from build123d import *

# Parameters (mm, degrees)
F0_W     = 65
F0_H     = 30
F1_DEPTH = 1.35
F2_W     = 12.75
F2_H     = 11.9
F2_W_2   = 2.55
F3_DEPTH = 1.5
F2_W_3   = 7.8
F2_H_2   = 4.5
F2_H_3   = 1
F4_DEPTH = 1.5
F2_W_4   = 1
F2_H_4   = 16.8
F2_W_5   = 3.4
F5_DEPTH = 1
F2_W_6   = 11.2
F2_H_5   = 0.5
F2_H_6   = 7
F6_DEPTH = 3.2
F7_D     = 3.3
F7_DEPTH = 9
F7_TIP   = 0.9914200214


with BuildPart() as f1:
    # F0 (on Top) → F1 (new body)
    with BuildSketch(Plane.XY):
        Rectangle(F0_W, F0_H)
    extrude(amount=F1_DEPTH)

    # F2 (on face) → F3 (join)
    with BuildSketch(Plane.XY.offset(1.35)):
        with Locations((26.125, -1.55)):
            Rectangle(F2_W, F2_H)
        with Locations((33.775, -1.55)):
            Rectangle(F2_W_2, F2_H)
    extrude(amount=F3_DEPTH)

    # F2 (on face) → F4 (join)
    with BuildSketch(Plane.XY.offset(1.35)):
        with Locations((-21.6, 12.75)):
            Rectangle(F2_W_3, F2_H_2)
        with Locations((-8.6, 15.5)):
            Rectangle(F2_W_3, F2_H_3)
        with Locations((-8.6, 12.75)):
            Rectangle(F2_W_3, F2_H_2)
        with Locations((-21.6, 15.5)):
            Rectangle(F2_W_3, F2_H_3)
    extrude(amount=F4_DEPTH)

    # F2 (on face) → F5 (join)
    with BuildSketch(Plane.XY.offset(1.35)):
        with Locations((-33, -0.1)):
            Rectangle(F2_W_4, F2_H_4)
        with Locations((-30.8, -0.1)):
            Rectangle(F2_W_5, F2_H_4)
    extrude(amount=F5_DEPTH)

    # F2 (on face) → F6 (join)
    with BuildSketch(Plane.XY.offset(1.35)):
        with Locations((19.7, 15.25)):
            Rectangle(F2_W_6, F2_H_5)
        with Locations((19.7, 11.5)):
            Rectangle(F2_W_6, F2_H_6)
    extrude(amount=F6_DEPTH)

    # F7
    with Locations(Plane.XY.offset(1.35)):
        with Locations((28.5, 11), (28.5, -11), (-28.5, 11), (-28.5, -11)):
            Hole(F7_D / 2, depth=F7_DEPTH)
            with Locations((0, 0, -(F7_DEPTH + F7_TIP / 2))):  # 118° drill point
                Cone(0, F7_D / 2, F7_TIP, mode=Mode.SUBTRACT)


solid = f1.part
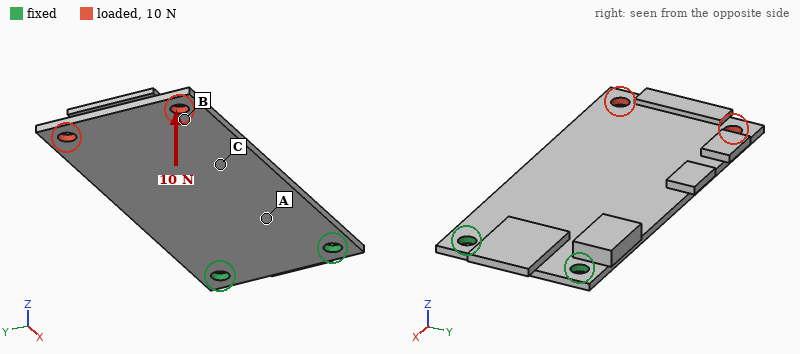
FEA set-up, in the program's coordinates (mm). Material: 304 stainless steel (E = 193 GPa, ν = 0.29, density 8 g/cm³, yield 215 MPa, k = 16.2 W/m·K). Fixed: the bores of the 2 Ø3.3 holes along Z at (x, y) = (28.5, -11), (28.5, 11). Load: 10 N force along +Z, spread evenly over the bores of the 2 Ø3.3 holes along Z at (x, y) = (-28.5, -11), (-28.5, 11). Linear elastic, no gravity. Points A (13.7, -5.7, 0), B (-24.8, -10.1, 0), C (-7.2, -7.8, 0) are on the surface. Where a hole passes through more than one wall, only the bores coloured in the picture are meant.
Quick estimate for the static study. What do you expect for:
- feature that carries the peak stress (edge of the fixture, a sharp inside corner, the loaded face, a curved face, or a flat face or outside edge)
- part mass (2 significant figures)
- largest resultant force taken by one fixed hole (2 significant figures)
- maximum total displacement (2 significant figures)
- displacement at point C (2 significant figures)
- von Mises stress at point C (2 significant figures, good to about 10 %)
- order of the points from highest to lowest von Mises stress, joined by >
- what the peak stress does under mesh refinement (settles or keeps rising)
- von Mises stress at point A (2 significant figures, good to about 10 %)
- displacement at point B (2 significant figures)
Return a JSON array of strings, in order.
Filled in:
["edge of the fixture", "27 g", "16 N", "0.40 mm", "0.15 mm", "21 MPa", "A > C > B", "keeps rising", "36 MPa", "0.32 mm"]
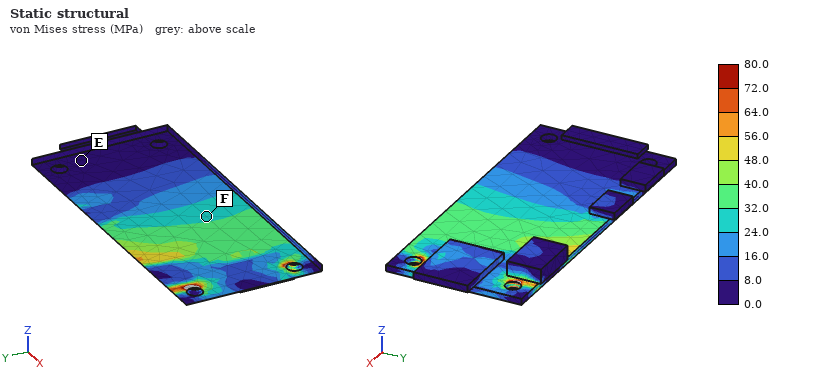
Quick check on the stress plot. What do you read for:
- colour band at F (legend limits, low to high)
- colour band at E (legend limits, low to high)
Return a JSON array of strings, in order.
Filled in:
["24.0 to 32.0 MPa", "0.0 to 8.0 MPa"]
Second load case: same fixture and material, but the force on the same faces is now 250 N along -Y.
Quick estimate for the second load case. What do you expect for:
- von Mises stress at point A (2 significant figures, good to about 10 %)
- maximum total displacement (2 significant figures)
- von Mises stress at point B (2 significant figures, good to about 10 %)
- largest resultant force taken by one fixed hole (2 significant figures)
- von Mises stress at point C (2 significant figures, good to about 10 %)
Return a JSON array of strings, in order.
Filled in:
["21 MPa", "40 µm", "15 MPa", "630 N", "17 MPa"]
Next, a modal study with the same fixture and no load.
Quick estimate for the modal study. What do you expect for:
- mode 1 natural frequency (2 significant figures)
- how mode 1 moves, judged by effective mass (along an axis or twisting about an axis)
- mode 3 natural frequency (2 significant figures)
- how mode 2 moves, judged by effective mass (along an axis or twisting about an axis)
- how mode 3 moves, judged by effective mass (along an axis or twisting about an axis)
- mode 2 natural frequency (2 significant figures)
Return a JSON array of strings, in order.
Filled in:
["330 Hz", "along Z", "2000 Hz", "twisting about X", "along Z", "1400 Hz"]
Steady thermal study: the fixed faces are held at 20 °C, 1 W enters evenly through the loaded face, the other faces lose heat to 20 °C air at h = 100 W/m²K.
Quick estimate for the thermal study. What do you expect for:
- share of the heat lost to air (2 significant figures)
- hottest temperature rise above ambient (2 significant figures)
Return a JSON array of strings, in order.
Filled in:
["100 %", "16 K"]
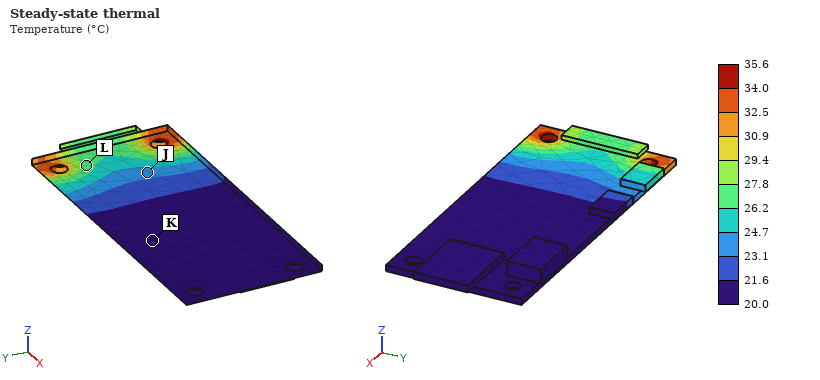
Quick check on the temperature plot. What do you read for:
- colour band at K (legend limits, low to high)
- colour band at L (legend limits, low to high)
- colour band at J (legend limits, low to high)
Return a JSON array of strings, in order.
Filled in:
["20.0 to 21.6 °C", "26.2 to 27.8 °C", "23.1 to 24.7 °C"]
